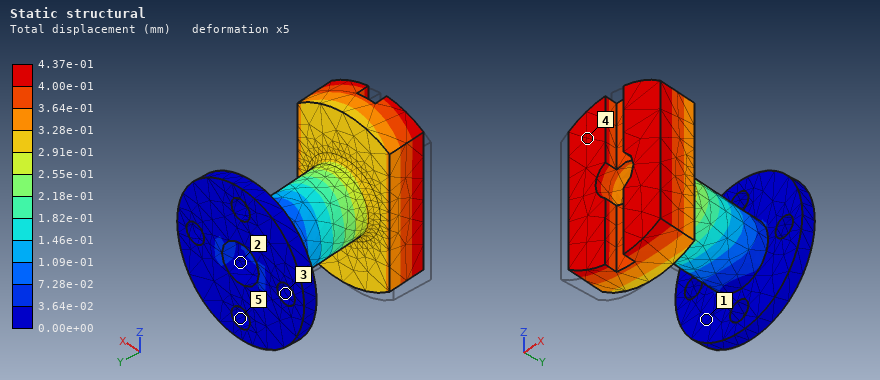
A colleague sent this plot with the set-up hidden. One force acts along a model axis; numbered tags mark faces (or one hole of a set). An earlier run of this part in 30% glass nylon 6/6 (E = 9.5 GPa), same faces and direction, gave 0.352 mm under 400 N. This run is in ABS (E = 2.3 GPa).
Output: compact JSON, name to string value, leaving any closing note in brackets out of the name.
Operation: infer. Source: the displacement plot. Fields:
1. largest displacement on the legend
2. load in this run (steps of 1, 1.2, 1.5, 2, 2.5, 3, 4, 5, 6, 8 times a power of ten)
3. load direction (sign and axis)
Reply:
{"largest displacement on the legend": "4.37e-01 mm", "load in this run": "120 N", "load direction": "+X"}
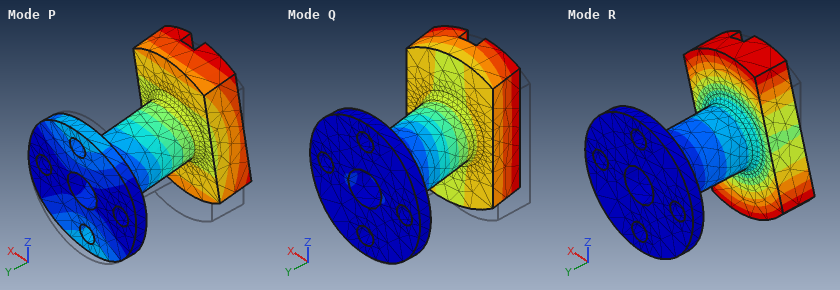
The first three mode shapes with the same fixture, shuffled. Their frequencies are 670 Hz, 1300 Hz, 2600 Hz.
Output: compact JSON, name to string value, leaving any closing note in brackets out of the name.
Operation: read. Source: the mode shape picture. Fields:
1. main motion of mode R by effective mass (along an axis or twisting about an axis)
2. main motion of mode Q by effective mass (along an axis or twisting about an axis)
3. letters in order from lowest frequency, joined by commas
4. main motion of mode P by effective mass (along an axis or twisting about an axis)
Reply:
{"main motion of mode R by effective mass": "twisting about Y", "main motion of mode Q by effective mass": "along X", "letters in order from lowest frequency, joined by commas": "P, Q, R", "main motion of mode P by effective mass": "along Z"}
